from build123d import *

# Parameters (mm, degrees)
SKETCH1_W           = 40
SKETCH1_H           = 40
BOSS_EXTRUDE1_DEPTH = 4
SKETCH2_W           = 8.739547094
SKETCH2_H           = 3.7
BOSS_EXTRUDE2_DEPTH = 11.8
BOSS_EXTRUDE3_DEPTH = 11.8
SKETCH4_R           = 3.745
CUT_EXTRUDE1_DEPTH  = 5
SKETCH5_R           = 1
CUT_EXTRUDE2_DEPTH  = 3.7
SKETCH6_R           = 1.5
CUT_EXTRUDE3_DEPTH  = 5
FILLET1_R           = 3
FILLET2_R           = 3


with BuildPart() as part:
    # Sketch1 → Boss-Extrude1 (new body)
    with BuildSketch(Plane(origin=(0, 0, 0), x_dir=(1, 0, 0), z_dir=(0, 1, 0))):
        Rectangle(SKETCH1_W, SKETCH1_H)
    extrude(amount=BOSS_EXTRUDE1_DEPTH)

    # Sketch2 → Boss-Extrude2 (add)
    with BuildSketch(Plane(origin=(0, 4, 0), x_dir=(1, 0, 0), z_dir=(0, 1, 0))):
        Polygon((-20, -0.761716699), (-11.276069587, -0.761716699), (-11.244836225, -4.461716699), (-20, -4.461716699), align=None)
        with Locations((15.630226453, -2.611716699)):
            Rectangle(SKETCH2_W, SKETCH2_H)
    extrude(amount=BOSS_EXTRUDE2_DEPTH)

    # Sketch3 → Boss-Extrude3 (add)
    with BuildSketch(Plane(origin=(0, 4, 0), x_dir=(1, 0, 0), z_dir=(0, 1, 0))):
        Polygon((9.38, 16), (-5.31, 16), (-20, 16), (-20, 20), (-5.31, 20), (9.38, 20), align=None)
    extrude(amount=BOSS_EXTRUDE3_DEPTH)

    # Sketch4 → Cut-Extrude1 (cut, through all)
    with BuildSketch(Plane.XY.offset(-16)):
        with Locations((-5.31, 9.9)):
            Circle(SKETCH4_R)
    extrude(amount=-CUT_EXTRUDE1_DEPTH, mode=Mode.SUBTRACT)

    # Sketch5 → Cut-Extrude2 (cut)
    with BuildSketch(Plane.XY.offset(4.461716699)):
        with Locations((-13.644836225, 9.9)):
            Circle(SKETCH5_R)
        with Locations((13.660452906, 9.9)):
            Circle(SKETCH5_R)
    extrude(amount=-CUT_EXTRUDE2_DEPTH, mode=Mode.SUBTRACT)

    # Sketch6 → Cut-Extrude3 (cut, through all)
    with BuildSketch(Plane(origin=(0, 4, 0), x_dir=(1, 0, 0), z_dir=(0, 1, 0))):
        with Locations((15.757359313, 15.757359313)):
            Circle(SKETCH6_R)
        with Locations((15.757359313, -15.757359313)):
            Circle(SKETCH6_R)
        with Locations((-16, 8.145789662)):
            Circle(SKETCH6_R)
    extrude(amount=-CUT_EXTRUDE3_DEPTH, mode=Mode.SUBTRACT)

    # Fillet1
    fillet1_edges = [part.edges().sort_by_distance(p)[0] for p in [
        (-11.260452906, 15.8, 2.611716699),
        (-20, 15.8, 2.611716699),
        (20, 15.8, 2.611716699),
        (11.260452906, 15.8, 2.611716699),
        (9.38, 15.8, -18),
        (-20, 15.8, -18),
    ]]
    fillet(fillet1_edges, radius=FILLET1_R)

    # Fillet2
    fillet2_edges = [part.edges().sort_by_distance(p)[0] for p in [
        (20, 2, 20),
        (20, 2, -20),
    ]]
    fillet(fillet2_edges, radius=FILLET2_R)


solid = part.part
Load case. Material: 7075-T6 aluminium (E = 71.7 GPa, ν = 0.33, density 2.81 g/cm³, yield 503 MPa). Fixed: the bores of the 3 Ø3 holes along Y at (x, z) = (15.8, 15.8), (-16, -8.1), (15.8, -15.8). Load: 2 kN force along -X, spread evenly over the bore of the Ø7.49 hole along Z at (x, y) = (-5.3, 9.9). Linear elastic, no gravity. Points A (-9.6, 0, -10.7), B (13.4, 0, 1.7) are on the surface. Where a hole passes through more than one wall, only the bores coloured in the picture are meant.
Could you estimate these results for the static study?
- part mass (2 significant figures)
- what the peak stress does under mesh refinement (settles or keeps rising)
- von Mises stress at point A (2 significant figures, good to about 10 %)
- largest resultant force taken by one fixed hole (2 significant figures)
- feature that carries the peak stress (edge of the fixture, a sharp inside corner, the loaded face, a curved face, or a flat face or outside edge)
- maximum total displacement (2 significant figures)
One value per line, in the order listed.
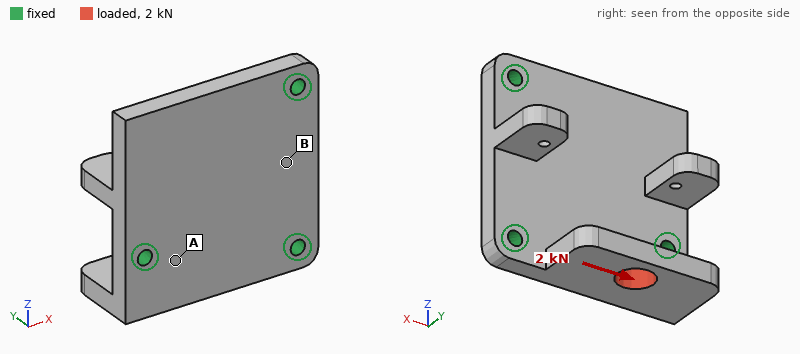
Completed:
23 g
keeps rising
25 MPa
1.1 kN
edge of the fixture
63 µm
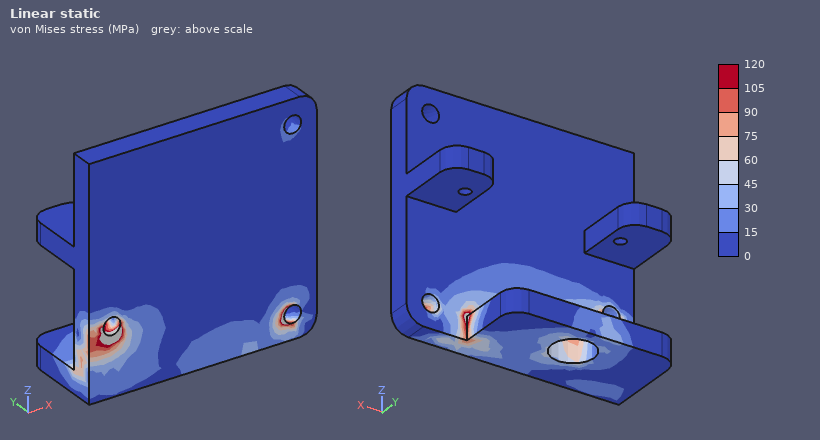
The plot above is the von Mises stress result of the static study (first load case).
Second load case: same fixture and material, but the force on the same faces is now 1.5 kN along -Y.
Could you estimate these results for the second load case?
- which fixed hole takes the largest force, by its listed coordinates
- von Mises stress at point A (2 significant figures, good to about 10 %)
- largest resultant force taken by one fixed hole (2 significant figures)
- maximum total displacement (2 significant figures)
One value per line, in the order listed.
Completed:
(-16, -8.1)
63 MPa
970 N
0.10 mm
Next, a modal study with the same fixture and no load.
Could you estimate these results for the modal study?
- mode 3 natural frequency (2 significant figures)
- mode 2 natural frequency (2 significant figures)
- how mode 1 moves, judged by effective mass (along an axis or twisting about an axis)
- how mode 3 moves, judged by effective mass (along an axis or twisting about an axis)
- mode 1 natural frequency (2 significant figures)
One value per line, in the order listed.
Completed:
13 kHz
8800 Hz
along Y
along Y
5900 Hz
